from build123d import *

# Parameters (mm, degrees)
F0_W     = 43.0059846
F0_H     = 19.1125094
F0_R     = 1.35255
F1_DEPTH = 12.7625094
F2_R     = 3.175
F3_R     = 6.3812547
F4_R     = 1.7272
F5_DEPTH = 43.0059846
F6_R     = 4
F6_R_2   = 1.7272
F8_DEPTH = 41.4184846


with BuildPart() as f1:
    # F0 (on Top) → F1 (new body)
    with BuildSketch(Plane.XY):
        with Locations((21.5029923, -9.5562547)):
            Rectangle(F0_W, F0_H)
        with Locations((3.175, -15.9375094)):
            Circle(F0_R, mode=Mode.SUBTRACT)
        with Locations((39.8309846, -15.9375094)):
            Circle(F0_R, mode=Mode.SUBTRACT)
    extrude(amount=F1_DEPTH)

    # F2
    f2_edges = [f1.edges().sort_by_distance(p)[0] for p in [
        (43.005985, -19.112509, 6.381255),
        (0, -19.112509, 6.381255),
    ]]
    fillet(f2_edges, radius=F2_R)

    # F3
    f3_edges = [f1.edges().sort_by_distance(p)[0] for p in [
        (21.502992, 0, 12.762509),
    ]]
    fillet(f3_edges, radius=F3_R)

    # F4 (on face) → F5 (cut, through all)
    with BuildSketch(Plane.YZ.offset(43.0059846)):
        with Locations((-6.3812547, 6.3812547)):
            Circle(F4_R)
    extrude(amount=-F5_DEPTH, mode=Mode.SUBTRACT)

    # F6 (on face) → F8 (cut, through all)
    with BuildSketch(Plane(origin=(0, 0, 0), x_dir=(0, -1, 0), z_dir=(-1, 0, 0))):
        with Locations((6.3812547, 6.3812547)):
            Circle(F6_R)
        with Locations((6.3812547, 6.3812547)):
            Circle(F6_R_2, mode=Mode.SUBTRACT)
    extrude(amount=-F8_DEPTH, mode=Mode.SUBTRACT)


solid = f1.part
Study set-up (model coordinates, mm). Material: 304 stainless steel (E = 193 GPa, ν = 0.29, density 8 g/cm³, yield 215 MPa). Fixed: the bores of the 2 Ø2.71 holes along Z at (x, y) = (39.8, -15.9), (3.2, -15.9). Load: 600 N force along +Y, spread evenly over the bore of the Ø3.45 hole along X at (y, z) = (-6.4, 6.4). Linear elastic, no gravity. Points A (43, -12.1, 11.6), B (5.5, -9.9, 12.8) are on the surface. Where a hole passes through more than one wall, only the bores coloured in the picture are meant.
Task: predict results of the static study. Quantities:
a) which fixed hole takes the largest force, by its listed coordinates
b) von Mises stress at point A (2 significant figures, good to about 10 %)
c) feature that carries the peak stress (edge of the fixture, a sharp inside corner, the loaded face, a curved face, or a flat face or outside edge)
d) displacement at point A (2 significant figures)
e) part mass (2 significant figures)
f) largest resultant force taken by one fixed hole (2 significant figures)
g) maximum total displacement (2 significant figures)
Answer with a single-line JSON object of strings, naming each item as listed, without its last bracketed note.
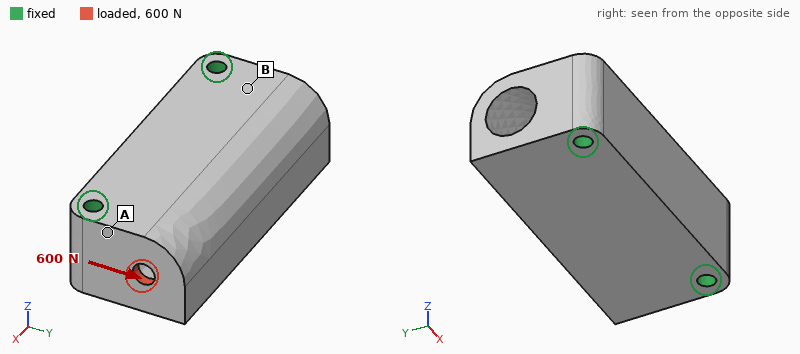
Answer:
{"which fixed hole takes the largest force, by its listed coordinates": "(39.8, -15.9)", "von Mises stress at point A": "12 MPa", "feature that carries the peak stress": "the loaded face", "displacement at point A": "0.28 µm", "part mass": "63 g", "largest resultant force taken by one fixed hole": "630 N", "maximum total displacement": "1.6 µm"}
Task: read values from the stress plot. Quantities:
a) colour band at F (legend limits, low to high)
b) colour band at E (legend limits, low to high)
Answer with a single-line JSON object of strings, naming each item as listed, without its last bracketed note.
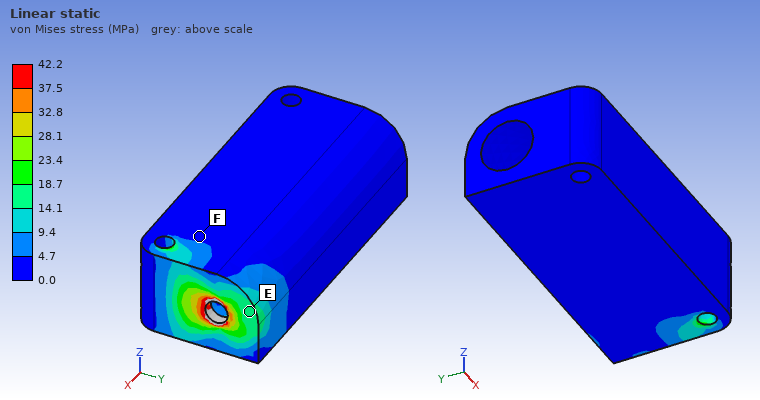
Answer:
{"colour band at F": "0.0 to 4.7 MPa", "colour band at E": "14.1 to 18.7 MPa"}
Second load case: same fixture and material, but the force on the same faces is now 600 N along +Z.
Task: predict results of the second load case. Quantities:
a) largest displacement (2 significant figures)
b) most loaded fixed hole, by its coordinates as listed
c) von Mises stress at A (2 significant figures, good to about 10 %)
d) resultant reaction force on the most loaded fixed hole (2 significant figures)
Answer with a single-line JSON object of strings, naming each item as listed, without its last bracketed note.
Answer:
{"largest displacement": "3.2 µm", "most loaded fixed hole, by its coordinates as listed": "(39.8, -15.9)", "von Mises stress at A": "17 MPa", "resultant reaction force on the most loaded fixed hole": "610 N"}
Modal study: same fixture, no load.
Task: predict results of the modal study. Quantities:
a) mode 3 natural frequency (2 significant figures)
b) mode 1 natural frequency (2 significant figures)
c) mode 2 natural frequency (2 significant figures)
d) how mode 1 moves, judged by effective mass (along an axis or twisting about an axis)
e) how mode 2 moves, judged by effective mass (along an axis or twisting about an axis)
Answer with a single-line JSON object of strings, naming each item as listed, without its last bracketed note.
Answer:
{"mode 3 natural frequency": "29 kHz", "mode 1 natural frequency": "17 kHz", "mode 2 natural frequency": "26 kHz", "how mode 1 moves, judged by effective mass": "along Z", "how mode 2 moves, judged by effective mass": "along Y"}
